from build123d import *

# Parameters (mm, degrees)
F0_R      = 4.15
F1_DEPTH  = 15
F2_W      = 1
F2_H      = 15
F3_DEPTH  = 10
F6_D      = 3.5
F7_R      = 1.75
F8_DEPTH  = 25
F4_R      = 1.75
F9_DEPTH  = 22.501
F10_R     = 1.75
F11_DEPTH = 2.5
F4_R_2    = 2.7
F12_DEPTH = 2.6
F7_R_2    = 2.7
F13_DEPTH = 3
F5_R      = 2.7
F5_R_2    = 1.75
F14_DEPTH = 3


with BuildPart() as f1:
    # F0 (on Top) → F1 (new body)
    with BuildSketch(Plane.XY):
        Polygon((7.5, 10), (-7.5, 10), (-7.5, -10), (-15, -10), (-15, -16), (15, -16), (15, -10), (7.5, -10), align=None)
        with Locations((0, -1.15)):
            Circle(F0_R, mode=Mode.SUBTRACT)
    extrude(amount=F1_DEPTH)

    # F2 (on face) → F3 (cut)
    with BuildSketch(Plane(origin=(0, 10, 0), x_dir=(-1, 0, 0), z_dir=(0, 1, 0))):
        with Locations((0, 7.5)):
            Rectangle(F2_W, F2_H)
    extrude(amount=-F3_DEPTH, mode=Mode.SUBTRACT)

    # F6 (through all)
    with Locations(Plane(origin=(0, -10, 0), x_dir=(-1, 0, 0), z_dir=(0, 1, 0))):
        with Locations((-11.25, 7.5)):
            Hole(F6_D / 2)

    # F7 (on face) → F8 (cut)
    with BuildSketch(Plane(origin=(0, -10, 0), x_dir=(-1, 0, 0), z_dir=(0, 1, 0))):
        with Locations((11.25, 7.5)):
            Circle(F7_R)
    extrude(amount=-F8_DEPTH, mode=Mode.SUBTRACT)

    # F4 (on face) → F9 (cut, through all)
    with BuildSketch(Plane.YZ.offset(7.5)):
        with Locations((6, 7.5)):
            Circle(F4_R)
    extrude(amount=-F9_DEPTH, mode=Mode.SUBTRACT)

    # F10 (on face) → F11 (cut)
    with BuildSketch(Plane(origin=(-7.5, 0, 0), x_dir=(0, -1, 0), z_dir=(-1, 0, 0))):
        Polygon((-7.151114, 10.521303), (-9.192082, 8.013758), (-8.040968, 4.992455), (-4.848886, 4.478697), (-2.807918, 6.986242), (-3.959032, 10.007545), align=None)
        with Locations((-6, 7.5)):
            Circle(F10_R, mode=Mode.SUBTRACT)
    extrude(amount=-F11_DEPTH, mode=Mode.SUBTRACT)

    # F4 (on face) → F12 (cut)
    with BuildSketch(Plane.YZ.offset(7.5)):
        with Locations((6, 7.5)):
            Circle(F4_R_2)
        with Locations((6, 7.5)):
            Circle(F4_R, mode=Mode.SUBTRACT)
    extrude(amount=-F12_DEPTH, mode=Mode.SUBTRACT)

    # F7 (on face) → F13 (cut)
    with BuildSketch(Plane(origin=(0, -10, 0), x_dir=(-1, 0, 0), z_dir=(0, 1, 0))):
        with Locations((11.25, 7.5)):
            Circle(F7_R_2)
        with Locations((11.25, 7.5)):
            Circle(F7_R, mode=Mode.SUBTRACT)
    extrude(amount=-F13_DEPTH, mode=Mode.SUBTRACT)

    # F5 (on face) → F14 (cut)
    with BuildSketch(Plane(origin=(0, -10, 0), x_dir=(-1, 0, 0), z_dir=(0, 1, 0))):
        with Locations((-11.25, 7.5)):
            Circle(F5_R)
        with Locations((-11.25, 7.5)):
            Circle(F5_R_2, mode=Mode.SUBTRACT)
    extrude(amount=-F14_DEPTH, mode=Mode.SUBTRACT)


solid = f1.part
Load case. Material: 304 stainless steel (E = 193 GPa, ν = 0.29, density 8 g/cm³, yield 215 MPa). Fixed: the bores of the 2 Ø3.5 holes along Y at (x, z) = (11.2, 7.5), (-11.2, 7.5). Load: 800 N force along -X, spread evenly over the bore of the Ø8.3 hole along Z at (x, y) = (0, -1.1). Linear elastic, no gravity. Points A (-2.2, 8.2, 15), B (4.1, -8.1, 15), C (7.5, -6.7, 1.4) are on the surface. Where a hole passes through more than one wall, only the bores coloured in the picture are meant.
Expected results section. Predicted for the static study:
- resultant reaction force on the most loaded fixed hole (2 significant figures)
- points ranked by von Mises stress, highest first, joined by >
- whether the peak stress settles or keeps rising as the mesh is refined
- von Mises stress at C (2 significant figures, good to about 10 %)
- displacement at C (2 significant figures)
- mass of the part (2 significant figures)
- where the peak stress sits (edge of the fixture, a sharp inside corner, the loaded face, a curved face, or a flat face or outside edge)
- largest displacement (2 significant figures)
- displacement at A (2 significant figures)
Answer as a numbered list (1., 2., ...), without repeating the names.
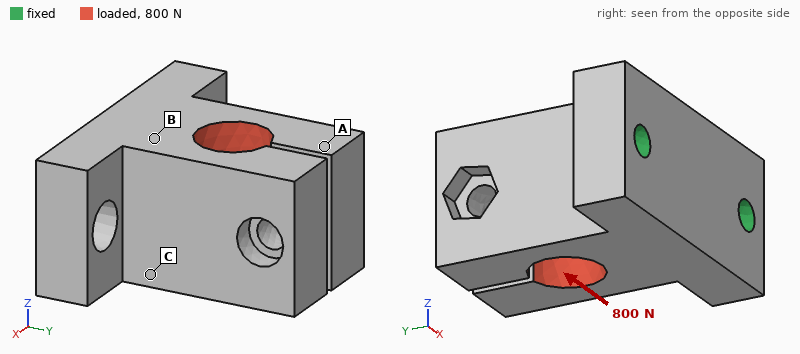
1. 640 N
2. C > B > A
3. keeps rising
4. 18 MPa
5. 1.6 µm
6. 47 g
7. edge of the fixture
8. 9.9 µm
9. 8.7 µm
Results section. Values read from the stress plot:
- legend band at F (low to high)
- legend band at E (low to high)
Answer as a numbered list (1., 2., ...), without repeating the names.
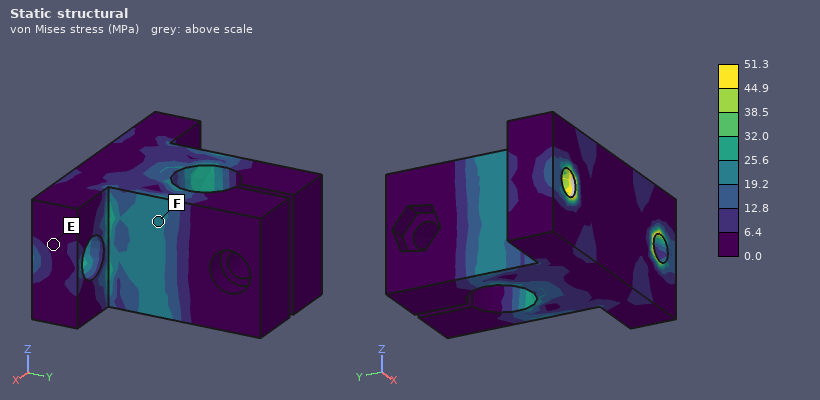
1. 19.2 to 25.6 MPa
2. 0.0 to 6.4 MPa
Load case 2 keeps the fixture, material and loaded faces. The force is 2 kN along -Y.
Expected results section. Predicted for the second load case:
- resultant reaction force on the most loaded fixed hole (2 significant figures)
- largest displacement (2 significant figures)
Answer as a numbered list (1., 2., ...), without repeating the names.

1. 1.1 kN
2. 15 µm
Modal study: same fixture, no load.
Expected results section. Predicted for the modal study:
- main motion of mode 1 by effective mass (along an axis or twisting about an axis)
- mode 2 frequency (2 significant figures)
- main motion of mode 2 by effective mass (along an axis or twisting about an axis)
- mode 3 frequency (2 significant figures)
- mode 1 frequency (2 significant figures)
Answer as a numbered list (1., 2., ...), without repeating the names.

1. along Z
2. 8000 Hz
3. along X
4. 8500 Hz
5. 5400 Hz
